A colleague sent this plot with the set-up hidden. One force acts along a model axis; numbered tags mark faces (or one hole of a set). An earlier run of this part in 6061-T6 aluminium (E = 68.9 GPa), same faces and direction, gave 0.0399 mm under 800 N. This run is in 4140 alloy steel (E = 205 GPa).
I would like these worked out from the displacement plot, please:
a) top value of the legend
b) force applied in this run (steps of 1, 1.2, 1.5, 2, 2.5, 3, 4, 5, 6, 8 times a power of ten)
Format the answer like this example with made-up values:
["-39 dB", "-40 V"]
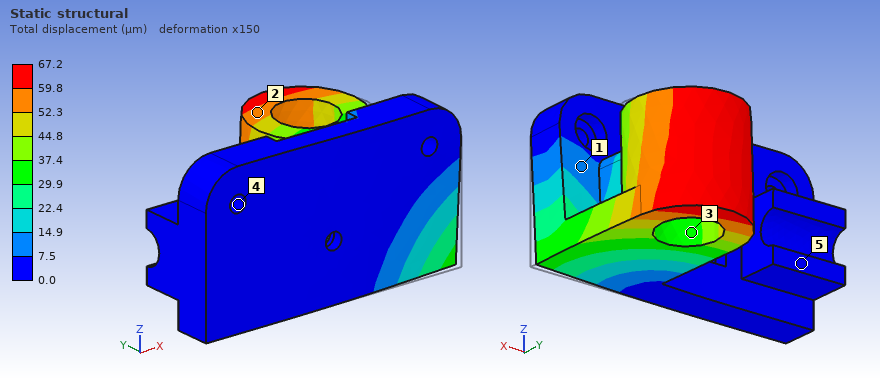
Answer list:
["67.2 µm", "4 kN"]
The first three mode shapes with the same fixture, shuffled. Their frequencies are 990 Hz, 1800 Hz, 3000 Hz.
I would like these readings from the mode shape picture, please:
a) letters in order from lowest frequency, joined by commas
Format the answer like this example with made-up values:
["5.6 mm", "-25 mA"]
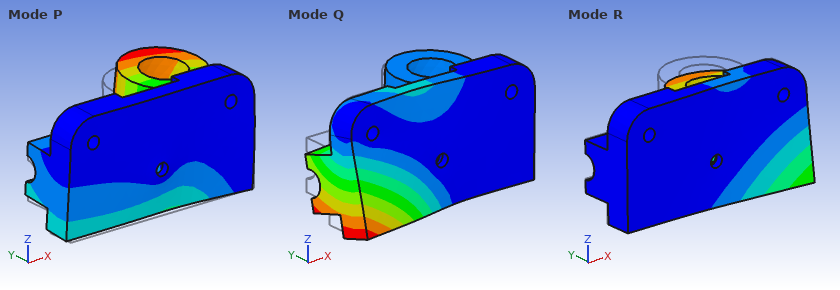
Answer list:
["R, P, Q"]
